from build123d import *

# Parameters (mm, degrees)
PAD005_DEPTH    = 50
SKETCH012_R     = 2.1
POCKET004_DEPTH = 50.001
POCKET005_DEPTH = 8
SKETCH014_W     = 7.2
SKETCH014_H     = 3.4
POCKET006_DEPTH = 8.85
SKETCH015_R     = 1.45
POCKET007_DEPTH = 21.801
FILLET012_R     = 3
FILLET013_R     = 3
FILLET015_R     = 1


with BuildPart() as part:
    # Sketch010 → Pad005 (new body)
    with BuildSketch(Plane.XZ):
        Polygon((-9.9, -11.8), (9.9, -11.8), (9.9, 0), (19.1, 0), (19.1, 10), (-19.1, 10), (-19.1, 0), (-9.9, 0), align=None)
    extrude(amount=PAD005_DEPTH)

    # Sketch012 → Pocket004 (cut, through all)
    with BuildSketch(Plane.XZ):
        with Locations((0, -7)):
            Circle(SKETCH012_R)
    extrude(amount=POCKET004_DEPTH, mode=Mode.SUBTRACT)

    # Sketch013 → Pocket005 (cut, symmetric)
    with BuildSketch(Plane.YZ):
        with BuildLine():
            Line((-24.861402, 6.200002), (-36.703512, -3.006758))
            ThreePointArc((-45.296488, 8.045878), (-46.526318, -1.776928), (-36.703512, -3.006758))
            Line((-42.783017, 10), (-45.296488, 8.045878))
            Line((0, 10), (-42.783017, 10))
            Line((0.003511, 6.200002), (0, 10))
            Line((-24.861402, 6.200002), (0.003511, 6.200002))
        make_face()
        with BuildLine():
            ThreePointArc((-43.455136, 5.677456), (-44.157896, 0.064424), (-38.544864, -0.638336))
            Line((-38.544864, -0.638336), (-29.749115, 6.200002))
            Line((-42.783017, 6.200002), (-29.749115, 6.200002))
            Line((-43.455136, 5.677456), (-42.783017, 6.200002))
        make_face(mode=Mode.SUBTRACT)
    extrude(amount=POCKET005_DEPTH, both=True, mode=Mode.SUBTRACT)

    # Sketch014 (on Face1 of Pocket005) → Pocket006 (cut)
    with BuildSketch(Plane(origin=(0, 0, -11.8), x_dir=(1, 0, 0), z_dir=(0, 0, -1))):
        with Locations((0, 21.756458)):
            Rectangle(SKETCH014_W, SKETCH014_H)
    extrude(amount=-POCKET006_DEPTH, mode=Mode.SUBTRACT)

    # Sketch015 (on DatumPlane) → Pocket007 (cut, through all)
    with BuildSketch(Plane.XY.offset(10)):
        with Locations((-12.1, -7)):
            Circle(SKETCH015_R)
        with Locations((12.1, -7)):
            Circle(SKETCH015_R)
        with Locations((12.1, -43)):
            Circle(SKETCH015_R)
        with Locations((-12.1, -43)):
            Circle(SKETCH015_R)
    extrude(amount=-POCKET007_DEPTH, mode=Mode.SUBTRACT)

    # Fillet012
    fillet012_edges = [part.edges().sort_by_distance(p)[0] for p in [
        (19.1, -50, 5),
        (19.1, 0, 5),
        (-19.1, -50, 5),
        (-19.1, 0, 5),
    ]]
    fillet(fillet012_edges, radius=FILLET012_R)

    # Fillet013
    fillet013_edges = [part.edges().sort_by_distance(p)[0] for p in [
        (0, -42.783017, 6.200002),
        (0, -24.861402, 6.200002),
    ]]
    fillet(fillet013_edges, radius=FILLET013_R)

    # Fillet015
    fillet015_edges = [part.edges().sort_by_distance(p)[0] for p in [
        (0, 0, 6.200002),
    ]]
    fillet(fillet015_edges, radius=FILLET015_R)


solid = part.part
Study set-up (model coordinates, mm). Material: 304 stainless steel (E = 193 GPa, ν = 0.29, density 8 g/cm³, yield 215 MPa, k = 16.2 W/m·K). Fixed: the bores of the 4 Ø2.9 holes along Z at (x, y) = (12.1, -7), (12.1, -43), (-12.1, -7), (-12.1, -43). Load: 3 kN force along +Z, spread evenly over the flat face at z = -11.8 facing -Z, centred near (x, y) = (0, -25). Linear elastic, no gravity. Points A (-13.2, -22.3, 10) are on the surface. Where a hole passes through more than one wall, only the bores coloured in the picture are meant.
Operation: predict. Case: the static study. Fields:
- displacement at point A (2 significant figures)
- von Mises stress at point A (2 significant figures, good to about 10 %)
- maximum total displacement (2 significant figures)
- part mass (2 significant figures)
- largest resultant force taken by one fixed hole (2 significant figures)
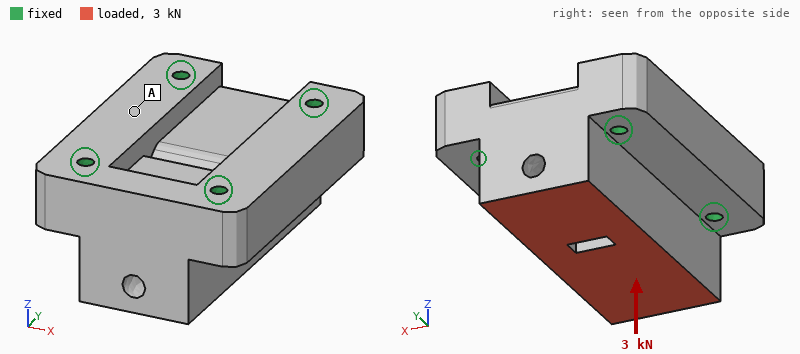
0.78 µm
4.1 MPa
1.4 µm
200 g
820 N
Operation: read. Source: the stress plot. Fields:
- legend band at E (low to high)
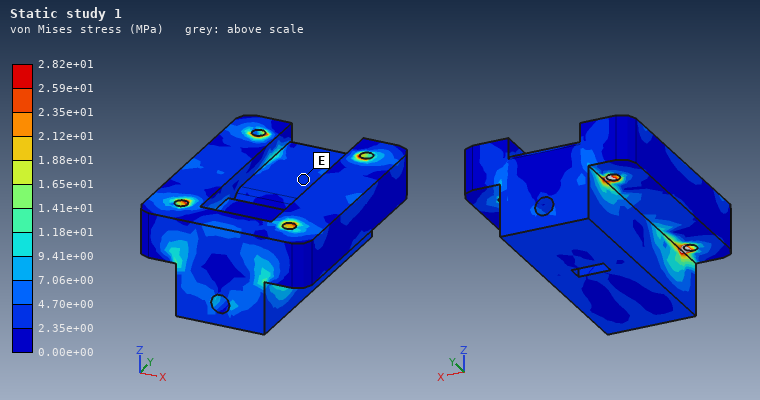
2.35e+00 to 4.70e+00 MPa
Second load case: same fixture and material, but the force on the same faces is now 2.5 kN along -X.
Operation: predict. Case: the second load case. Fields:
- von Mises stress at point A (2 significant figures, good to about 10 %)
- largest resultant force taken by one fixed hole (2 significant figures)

4.1 MPa
1.2 kN
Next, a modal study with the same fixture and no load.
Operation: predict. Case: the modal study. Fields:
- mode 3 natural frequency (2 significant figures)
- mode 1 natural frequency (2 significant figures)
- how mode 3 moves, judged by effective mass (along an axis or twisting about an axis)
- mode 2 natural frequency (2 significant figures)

26 kHz
22 kHz
along Y
22 kHz
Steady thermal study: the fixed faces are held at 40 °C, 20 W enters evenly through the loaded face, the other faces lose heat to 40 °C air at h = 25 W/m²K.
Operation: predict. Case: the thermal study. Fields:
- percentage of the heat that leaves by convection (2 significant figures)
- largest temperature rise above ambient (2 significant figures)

15 %
40 K
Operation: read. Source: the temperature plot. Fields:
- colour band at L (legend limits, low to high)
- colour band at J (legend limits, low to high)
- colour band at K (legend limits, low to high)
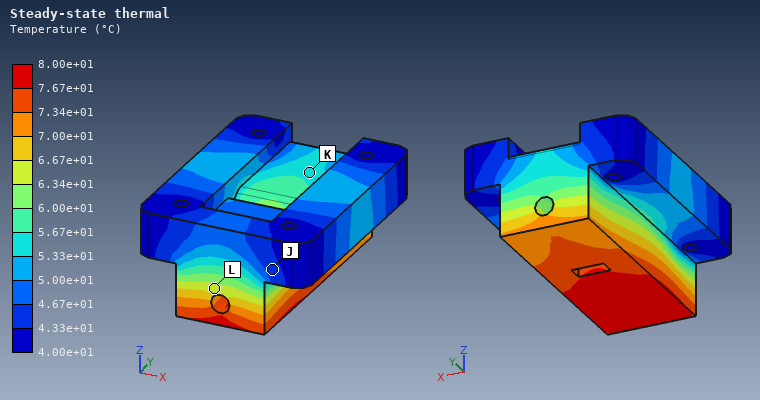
6.34e+01 to 6.67e+01 °C
4.33e+01 to 4.67e+01 °C
5.33e+01 to 5.67e+01 °C
